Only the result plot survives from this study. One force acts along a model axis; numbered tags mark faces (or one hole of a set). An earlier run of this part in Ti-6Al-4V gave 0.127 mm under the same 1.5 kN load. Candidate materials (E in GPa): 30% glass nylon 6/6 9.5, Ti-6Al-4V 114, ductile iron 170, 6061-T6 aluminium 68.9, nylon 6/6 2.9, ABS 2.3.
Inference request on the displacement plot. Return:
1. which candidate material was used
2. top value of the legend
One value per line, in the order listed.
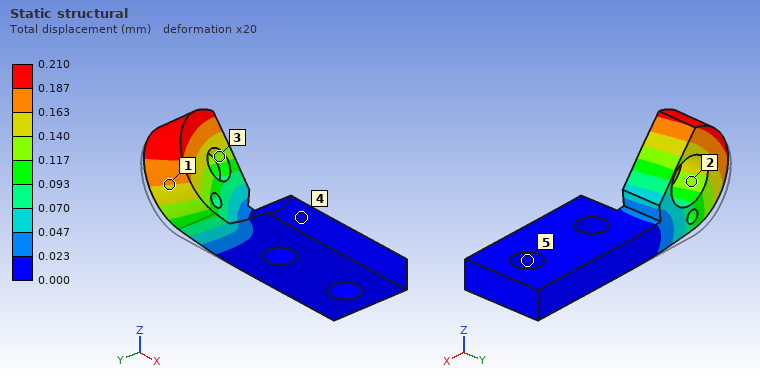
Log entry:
6061-T6 aluminium
0.210 mm
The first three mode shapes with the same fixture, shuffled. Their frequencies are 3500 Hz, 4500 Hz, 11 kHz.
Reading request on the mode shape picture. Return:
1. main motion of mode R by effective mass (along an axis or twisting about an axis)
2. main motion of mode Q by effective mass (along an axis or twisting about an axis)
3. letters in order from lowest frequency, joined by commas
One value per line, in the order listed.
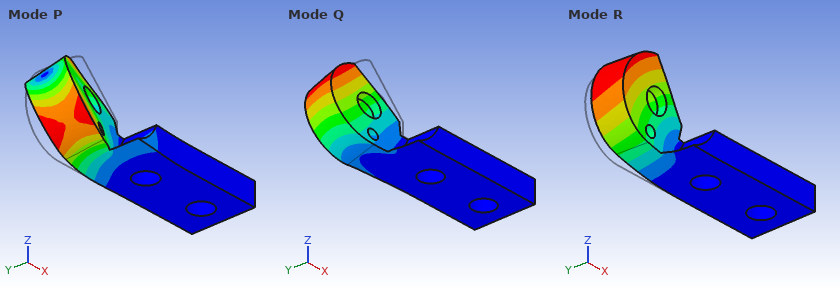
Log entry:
along Z
along Y
R, Q, P
